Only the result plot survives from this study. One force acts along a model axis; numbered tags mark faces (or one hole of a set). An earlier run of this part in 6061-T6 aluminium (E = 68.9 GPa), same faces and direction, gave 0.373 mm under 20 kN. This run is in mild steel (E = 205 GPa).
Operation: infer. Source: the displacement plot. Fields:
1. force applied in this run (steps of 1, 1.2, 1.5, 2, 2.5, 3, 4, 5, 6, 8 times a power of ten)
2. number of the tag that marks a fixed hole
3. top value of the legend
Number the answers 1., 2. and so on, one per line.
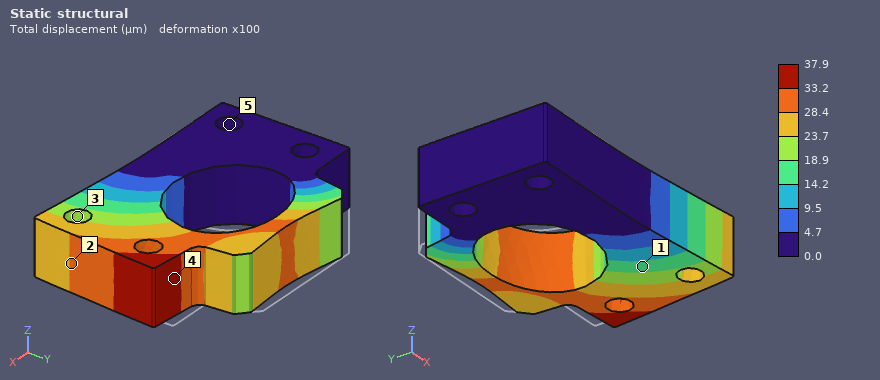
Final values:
1. 6 kN
2. 5
3. 37.9 µm
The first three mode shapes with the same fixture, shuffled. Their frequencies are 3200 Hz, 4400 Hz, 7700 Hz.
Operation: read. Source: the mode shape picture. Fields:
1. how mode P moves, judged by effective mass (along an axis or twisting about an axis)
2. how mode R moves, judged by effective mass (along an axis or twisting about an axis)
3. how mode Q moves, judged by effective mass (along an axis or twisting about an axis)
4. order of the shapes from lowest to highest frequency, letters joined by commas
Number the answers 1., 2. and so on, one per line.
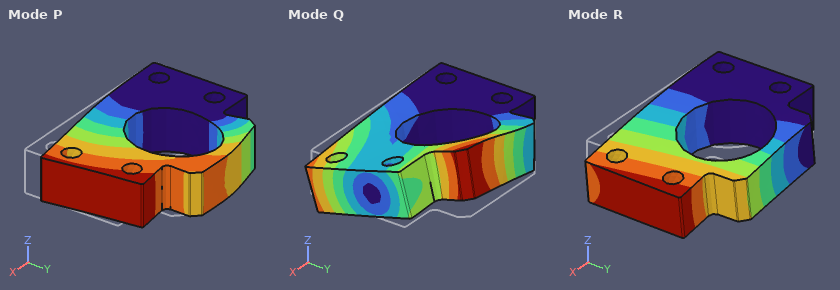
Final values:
1. along Y
2. along Z
3. twisting about X
4. R, P, Q
